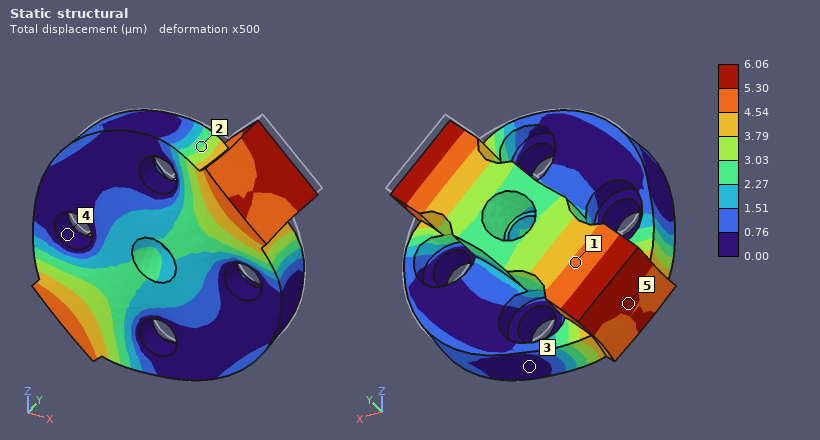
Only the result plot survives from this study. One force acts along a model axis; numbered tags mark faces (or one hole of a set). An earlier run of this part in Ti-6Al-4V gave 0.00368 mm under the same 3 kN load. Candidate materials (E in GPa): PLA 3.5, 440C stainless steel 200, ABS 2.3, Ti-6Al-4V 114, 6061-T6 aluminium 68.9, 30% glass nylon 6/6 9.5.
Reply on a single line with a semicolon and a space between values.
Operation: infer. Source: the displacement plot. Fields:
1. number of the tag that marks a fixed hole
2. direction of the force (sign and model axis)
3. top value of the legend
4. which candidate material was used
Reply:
4; -Y; 6.06 µm; 6061-T6 aluminium
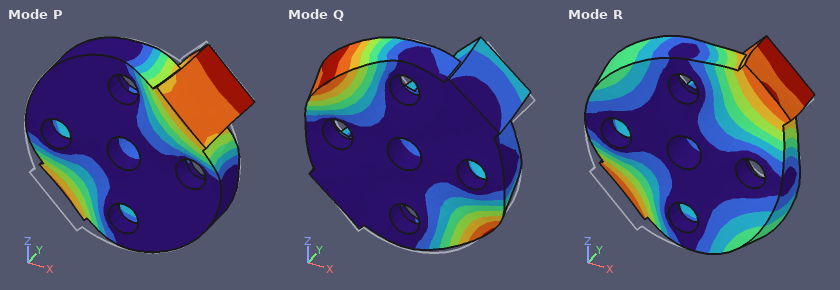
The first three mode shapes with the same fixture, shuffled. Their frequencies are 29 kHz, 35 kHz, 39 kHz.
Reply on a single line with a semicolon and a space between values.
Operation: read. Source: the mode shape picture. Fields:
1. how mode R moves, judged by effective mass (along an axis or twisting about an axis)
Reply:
along Y
